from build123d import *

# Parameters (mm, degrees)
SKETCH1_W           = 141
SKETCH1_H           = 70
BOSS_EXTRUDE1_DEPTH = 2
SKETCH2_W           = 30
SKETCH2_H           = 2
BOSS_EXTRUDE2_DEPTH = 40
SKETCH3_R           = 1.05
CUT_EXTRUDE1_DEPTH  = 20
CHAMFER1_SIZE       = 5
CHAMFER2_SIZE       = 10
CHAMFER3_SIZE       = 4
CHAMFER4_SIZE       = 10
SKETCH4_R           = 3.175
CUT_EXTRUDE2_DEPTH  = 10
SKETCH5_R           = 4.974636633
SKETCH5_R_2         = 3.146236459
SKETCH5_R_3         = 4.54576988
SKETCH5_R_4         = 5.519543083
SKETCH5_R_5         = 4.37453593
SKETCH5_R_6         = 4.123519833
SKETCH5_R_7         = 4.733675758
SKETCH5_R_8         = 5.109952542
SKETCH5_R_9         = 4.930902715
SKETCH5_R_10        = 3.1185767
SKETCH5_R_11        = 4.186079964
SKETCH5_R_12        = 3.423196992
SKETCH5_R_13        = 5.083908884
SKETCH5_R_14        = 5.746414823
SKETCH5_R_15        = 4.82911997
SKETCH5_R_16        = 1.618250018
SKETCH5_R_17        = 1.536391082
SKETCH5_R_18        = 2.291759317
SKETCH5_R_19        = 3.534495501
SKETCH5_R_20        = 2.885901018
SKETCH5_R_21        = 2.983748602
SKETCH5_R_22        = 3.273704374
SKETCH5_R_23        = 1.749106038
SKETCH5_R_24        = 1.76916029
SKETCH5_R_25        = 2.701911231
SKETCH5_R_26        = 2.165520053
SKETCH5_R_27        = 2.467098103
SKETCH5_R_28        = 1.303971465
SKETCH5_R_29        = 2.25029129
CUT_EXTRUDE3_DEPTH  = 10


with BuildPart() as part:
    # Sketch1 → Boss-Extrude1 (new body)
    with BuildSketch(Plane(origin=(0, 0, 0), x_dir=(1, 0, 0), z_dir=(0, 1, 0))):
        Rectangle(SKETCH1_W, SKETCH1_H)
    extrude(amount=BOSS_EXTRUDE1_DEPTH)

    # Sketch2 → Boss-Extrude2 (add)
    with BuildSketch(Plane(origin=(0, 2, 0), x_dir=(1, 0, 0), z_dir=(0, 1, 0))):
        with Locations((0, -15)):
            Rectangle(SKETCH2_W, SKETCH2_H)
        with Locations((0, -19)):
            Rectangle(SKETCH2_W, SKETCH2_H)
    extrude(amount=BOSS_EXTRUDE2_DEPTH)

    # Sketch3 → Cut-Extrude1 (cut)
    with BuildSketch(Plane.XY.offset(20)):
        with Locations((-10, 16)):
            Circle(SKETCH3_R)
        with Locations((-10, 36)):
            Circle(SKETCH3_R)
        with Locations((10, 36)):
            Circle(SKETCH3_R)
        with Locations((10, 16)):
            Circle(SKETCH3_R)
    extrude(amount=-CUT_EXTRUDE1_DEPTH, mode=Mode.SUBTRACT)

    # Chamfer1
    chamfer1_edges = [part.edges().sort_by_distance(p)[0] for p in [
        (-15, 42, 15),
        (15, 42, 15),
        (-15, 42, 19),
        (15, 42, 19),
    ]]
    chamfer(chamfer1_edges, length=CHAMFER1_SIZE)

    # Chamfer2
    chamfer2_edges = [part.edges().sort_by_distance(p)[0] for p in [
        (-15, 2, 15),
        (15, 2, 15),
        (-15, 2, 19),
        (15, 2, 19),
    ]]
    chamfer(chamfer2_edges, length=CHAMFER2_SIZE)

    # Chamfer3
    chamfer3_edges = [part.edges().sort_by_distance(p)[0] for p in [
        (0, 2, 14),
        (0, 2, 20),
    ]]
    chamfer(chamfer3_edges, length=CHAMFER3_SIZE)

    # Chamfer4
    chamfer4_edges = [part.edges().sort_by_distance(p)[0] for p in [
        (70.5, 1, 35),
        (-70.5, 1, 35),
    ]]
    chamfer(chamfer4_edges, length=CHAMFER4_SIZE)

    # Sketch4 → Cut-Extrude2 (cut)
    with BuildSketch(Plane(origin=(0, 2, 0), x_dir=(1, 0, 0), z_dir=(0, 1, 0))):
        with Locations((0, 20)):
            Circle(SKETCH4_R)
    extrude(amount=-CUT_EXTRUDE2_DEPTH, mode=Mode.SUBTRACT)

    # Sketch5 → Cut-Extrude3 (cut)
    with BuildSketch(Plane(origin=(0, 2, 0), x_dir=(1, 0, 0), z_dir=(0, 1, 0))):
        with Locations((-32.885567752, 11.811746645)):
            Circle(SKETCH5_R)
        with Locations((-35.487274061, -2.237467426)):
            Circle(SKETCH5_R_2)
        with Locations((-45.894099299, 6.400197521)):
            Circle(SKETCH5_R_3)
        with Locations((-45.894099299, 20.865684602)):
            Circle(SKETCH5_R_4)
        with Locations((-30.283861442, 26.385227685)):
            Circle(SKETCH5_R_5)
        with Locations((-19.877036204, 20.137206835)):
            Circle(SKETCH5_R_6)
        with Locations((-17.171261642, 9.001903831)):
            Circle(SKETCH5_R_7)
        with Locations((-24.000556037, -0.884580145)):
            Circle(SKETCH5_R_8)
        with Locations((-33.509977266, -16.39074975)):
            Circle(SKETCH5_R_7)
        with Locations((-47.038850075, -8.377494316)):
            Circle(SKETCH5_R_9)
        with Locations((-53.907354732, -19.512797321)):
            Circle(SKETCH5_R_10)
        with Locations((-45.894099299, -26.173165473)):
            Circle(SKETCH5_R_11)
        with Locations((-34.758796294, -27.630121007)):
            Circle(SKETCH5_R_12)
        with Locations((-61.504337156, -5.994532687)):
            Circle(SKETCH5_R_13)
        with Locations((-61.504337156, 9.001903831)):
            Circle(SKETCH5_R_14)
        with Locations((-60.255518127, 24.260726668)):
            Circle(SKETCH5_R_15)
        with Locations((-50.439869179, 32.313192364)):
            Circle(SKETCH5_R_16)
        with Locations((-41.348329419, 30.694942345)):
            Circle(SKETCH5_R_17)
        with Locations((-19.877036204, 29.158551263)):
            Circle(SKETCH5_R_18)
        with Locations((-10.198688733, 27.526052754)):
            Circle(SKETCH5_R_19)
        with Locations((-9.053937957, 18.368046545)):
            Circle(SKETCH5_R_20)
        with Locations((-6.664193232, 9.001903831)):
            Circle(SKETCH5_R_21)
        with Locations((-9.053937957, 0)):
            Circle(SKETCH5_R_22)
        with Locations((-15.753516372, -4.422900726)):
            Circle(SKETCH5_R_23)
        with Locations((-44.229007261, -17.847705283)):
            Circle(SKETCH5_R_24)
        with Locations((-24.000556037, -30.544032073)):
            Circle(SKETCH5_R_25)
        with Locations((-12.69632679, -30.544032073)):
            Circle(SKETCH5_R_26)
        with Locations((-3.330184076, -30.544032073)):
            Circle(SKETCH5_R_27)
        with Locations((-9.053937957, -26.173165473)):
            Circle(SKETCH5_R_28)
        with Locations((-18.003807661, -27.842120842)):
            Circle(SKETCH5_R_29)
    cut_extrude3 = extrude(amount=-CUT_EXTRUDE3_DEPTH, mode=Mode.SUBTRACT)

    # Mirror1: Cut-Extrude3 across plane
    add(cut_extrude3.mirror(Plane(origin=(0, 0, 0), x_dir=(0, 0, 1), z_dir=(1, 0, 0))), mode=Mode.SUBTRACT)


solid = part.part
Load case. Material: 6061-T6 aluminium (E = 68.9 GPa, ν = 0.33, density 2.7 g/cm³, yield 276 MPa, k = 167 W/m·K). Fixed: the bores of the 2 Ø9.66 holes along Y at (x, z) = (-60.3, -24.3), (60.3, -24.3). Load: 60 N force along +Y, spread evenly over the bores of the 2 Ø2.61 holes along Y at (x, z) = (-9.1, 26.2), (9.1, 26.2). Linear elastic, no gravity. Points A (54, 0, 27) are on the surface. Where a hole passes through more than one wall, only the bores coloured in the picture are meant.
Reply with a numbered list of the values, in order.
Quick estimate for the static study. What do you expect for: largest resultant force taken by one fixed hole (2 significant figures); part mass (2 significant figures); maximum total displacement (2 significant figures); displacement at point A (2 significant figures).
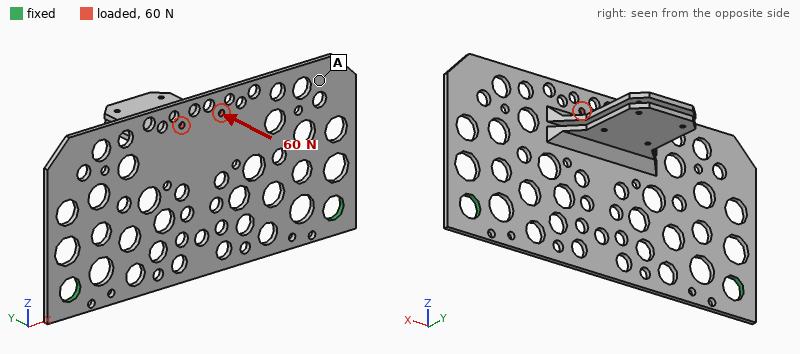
1. 30 N
2. 54 g
3. 1.5 mm
4. 0.98 mm
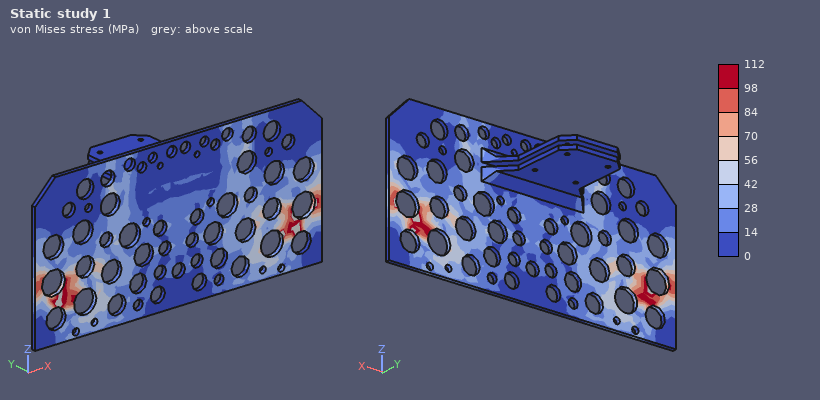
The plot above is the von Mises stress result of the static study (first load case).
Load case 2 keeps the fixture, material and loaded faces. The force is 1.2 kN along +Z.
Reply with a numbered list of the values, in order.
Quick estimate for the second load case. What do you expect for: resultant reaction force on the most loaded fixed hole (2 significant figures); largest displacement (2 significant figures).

1. 690 N
2. 42 µm
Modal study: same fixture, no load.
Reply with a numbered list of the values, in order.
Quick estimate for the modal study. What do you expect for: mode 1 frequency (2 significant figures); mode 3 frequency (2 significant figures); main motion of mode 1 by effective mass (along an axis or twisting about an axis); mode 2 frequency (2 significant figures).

1. 220 Hz
2. 630 Hz
3. along Y
4. 610 Hz
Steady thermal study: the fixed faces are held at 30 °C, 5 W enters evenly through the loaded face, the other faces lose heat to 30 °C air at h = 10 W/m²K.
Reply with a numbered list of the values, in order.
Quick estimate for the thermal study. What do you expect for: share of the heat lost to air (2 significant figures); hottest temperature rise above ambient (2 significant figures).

1. 36 %
2. 16 K
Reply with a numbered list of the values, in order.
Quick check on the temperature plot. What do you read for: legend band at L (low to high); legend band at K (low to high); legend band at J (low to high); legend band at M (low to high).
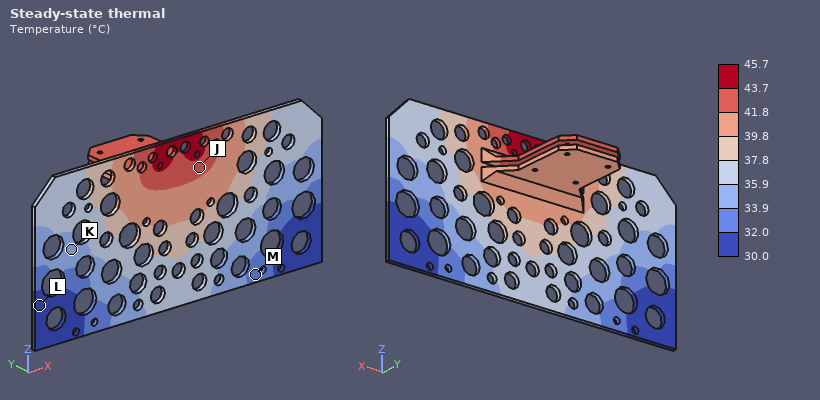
1. 30.0 to 32.0 °C
2. 33.9 to 35.9 °C
3. 41.8 to 43.7 °C
4. 32.0 to 33.9 °C
